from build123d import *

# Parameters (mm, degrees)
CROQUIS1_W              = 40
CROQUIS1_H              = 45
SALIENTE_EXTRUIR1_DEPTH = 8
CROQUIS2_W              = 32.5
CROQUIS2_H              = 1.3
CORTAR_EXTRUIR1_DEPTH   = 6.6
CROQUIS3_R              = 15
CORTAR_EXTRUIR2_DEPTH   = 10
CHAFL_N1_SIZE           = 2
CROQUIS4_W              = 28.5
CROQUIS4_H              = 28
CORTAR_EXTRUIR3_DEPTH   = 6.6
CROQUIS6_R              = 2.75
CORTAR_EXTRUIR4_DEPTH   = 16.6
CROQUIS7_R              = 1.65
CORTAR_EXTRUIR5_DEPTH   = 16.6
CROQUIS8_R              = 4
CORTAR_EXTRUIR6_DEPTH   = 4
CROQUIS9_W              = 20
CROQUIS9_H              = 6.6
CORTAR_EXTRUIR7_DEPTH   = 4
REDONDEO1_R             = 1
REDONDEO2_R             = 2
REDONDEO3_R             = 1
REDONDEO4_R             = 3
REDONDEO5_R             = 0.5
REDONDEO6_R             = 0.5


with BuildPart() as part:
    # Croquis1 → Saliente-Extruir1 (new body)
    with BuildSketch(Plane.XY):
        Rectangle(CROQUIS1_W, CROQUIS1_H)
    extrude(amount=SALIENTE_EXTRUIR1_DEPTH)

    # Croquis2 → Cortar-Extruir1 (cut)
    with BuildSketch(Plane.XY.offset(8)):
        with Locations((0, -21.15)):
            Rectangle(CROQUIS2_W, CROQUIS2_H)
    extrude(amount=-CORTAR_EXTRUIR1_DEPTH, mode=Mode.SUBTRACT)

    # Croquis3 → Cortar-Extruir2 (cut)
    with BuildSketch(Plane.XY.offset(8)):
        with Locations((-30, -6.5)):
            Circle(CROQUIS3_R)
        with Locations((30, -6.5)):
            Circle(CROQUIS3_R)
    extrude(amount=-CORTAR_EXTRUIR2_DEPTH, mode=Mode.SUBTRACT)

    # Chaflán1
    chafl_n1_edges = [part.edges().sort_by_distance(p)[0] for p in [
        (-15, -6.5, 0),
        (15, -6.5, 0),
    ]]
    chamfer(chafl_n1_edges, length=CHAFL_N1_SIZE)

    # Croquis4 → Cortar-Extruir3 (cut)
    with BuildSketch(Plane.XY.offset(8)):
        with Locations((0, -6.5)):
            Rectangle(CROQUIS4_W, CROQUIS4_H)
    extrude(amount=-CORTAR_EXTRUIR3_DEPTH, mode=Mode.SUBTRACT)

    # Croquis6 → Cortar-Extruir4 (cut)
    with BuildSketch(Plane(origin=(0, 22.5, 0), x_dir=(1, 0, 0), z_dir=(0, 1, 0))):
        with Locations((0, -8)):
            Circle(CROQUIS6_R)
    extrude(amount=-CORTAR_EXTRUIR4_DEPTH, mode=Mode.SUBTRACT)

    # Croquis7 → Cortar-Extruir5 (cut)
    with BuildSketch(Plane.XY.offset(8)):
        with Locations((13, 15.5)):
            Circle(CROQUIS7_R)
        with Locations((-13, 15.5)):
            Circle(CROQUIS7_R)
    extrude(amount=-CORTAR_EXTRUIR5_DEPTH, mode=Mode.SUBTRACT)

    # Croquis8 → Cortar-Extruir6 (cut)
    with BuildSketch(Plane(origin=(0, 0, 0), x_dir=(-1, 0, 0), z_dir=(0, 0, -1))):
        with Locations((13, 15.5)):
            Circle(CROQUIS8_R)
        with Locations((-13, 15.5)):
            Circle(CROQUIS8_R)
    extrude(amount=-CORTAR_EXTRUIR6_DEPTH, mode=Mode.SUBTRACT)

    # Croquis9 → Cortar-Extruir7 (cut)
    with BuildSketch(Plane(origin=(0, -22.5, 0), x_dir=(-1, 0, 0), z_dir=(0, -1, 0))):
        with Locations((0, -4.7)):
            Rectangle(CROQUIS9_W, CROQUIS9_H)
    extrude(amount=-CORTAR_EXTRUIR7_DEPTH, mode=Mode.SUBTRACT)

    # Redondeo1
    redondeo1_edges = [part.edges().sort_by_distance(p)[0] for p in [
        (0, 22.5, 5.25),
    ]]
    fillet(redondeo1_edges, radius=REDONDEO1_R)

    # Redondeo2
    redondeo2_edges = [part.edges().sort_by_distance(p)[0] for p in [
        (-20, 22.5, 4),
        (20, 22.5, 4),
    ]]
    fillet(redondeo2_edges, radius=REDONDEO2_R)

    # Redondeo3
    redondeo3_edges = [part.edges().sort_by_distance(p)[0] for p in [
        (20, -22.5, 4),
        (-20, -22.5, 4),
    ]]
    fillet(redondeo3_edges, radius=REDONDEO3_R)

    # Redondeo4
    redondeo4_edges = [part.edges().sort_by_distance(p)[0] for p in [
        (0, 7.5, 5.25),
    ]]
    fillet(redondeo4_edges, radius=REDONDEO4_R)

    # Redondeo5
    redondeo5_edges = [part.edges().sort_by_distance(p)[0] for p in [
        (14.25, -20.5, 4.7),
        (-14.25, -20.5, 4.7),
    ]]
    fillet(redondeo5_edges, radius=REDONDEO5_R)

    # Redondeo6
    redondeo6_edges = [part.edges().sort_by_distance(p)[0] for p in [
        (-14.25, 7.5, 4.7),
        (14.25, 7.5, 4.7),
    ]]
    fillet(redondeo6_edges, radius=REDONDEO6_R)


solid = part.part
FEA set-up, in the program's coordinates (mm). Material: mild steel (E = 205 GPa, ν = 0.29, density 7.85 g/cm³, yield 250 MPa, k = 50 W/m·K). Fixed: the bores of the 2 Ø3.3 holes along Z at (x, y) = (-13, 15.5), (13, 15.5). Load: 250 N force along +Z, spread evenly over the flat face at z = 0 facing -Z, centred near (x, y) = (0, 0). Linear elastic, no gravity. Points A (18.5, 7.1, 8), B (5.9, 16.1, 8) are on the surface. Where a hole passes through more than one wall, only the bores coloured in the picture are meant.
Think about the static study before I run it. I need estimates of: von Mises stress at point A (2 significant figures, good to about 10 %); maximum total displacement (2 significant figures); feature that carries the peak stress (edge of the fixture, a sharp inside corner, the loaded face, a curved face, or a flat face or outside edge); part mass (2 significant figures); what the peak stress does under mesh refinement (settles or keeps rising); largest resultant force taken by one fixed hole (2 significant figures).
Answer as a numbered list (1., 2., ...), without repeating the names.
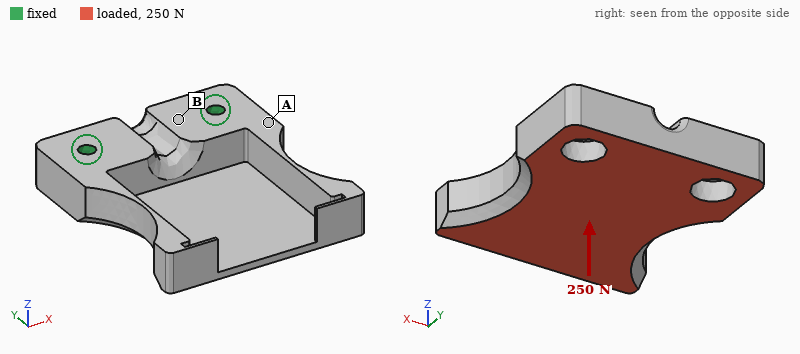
1. 15 MPa
2. 41 µm
3. edge of the fixture
4. 53 g
5. keeps rising
6. 130 N
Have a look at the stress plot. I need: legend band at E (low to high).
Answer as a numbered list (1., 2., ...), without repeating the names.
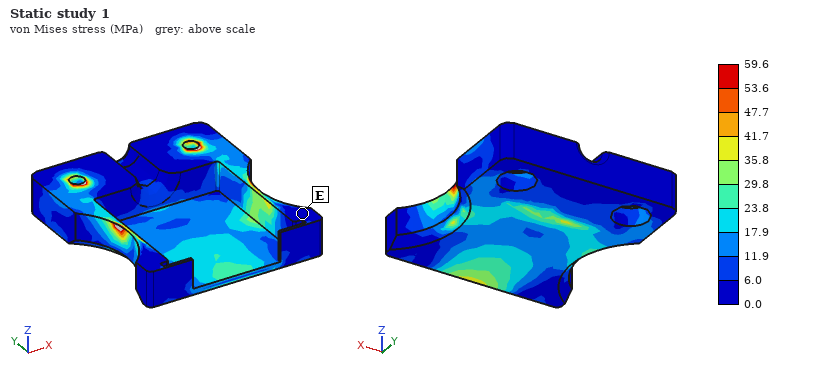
1. 0.0 to 6.0 MPa
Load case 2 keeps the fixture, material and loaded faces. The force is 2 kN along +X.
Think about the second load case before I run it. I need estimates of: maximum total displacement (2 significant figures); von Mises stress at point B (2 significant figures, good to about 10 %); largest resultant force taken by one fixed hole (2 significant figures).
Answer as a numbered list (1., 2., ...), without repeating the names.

1. 30 µm
2. 15 MPa
3. 1.5 kN
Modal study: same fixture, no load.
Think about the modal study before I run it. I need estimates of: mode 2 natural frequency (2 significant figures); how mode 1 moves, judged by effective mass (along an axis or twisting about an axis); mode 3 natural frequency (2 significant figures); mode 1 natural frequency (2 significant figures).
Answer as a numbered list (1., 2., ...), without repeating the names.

1. 3500 Hz
2. along Z
3. 4500 Hz
4. 3300 Hz
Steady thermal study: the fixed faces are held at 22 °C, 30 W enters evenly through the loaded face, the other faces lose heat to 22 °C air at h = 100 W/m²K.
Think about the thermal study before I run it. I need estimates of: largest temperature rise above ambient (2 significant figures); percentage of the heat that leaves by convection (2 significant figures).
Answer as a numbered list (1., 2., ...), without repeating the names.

1. 63 K
2. 37 %
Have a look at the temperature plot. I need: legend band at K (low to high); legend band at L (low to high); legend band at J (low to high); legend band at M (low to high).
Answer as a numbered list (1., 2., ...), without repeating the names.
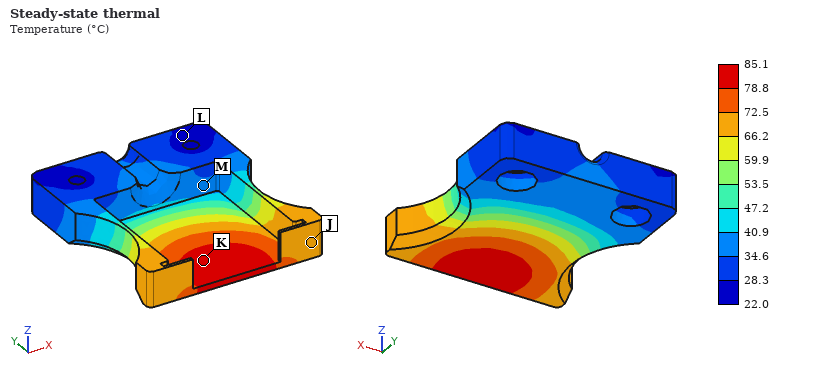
1. 78.8 to 85.1 °C
2. 22.0 to 28.3 °C
3. 66.2 to 72.5 °C
4. 34.6 to 40.9 °C
